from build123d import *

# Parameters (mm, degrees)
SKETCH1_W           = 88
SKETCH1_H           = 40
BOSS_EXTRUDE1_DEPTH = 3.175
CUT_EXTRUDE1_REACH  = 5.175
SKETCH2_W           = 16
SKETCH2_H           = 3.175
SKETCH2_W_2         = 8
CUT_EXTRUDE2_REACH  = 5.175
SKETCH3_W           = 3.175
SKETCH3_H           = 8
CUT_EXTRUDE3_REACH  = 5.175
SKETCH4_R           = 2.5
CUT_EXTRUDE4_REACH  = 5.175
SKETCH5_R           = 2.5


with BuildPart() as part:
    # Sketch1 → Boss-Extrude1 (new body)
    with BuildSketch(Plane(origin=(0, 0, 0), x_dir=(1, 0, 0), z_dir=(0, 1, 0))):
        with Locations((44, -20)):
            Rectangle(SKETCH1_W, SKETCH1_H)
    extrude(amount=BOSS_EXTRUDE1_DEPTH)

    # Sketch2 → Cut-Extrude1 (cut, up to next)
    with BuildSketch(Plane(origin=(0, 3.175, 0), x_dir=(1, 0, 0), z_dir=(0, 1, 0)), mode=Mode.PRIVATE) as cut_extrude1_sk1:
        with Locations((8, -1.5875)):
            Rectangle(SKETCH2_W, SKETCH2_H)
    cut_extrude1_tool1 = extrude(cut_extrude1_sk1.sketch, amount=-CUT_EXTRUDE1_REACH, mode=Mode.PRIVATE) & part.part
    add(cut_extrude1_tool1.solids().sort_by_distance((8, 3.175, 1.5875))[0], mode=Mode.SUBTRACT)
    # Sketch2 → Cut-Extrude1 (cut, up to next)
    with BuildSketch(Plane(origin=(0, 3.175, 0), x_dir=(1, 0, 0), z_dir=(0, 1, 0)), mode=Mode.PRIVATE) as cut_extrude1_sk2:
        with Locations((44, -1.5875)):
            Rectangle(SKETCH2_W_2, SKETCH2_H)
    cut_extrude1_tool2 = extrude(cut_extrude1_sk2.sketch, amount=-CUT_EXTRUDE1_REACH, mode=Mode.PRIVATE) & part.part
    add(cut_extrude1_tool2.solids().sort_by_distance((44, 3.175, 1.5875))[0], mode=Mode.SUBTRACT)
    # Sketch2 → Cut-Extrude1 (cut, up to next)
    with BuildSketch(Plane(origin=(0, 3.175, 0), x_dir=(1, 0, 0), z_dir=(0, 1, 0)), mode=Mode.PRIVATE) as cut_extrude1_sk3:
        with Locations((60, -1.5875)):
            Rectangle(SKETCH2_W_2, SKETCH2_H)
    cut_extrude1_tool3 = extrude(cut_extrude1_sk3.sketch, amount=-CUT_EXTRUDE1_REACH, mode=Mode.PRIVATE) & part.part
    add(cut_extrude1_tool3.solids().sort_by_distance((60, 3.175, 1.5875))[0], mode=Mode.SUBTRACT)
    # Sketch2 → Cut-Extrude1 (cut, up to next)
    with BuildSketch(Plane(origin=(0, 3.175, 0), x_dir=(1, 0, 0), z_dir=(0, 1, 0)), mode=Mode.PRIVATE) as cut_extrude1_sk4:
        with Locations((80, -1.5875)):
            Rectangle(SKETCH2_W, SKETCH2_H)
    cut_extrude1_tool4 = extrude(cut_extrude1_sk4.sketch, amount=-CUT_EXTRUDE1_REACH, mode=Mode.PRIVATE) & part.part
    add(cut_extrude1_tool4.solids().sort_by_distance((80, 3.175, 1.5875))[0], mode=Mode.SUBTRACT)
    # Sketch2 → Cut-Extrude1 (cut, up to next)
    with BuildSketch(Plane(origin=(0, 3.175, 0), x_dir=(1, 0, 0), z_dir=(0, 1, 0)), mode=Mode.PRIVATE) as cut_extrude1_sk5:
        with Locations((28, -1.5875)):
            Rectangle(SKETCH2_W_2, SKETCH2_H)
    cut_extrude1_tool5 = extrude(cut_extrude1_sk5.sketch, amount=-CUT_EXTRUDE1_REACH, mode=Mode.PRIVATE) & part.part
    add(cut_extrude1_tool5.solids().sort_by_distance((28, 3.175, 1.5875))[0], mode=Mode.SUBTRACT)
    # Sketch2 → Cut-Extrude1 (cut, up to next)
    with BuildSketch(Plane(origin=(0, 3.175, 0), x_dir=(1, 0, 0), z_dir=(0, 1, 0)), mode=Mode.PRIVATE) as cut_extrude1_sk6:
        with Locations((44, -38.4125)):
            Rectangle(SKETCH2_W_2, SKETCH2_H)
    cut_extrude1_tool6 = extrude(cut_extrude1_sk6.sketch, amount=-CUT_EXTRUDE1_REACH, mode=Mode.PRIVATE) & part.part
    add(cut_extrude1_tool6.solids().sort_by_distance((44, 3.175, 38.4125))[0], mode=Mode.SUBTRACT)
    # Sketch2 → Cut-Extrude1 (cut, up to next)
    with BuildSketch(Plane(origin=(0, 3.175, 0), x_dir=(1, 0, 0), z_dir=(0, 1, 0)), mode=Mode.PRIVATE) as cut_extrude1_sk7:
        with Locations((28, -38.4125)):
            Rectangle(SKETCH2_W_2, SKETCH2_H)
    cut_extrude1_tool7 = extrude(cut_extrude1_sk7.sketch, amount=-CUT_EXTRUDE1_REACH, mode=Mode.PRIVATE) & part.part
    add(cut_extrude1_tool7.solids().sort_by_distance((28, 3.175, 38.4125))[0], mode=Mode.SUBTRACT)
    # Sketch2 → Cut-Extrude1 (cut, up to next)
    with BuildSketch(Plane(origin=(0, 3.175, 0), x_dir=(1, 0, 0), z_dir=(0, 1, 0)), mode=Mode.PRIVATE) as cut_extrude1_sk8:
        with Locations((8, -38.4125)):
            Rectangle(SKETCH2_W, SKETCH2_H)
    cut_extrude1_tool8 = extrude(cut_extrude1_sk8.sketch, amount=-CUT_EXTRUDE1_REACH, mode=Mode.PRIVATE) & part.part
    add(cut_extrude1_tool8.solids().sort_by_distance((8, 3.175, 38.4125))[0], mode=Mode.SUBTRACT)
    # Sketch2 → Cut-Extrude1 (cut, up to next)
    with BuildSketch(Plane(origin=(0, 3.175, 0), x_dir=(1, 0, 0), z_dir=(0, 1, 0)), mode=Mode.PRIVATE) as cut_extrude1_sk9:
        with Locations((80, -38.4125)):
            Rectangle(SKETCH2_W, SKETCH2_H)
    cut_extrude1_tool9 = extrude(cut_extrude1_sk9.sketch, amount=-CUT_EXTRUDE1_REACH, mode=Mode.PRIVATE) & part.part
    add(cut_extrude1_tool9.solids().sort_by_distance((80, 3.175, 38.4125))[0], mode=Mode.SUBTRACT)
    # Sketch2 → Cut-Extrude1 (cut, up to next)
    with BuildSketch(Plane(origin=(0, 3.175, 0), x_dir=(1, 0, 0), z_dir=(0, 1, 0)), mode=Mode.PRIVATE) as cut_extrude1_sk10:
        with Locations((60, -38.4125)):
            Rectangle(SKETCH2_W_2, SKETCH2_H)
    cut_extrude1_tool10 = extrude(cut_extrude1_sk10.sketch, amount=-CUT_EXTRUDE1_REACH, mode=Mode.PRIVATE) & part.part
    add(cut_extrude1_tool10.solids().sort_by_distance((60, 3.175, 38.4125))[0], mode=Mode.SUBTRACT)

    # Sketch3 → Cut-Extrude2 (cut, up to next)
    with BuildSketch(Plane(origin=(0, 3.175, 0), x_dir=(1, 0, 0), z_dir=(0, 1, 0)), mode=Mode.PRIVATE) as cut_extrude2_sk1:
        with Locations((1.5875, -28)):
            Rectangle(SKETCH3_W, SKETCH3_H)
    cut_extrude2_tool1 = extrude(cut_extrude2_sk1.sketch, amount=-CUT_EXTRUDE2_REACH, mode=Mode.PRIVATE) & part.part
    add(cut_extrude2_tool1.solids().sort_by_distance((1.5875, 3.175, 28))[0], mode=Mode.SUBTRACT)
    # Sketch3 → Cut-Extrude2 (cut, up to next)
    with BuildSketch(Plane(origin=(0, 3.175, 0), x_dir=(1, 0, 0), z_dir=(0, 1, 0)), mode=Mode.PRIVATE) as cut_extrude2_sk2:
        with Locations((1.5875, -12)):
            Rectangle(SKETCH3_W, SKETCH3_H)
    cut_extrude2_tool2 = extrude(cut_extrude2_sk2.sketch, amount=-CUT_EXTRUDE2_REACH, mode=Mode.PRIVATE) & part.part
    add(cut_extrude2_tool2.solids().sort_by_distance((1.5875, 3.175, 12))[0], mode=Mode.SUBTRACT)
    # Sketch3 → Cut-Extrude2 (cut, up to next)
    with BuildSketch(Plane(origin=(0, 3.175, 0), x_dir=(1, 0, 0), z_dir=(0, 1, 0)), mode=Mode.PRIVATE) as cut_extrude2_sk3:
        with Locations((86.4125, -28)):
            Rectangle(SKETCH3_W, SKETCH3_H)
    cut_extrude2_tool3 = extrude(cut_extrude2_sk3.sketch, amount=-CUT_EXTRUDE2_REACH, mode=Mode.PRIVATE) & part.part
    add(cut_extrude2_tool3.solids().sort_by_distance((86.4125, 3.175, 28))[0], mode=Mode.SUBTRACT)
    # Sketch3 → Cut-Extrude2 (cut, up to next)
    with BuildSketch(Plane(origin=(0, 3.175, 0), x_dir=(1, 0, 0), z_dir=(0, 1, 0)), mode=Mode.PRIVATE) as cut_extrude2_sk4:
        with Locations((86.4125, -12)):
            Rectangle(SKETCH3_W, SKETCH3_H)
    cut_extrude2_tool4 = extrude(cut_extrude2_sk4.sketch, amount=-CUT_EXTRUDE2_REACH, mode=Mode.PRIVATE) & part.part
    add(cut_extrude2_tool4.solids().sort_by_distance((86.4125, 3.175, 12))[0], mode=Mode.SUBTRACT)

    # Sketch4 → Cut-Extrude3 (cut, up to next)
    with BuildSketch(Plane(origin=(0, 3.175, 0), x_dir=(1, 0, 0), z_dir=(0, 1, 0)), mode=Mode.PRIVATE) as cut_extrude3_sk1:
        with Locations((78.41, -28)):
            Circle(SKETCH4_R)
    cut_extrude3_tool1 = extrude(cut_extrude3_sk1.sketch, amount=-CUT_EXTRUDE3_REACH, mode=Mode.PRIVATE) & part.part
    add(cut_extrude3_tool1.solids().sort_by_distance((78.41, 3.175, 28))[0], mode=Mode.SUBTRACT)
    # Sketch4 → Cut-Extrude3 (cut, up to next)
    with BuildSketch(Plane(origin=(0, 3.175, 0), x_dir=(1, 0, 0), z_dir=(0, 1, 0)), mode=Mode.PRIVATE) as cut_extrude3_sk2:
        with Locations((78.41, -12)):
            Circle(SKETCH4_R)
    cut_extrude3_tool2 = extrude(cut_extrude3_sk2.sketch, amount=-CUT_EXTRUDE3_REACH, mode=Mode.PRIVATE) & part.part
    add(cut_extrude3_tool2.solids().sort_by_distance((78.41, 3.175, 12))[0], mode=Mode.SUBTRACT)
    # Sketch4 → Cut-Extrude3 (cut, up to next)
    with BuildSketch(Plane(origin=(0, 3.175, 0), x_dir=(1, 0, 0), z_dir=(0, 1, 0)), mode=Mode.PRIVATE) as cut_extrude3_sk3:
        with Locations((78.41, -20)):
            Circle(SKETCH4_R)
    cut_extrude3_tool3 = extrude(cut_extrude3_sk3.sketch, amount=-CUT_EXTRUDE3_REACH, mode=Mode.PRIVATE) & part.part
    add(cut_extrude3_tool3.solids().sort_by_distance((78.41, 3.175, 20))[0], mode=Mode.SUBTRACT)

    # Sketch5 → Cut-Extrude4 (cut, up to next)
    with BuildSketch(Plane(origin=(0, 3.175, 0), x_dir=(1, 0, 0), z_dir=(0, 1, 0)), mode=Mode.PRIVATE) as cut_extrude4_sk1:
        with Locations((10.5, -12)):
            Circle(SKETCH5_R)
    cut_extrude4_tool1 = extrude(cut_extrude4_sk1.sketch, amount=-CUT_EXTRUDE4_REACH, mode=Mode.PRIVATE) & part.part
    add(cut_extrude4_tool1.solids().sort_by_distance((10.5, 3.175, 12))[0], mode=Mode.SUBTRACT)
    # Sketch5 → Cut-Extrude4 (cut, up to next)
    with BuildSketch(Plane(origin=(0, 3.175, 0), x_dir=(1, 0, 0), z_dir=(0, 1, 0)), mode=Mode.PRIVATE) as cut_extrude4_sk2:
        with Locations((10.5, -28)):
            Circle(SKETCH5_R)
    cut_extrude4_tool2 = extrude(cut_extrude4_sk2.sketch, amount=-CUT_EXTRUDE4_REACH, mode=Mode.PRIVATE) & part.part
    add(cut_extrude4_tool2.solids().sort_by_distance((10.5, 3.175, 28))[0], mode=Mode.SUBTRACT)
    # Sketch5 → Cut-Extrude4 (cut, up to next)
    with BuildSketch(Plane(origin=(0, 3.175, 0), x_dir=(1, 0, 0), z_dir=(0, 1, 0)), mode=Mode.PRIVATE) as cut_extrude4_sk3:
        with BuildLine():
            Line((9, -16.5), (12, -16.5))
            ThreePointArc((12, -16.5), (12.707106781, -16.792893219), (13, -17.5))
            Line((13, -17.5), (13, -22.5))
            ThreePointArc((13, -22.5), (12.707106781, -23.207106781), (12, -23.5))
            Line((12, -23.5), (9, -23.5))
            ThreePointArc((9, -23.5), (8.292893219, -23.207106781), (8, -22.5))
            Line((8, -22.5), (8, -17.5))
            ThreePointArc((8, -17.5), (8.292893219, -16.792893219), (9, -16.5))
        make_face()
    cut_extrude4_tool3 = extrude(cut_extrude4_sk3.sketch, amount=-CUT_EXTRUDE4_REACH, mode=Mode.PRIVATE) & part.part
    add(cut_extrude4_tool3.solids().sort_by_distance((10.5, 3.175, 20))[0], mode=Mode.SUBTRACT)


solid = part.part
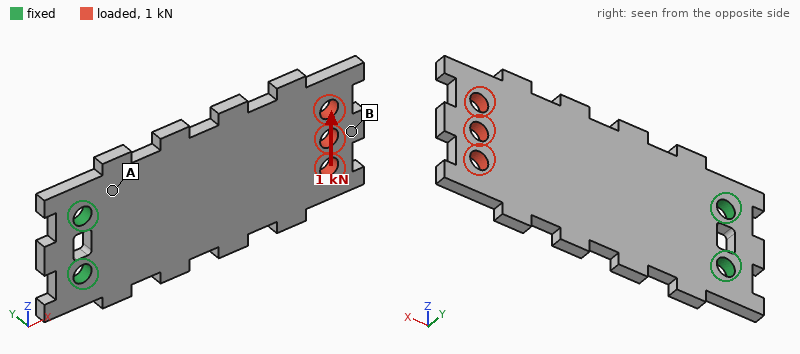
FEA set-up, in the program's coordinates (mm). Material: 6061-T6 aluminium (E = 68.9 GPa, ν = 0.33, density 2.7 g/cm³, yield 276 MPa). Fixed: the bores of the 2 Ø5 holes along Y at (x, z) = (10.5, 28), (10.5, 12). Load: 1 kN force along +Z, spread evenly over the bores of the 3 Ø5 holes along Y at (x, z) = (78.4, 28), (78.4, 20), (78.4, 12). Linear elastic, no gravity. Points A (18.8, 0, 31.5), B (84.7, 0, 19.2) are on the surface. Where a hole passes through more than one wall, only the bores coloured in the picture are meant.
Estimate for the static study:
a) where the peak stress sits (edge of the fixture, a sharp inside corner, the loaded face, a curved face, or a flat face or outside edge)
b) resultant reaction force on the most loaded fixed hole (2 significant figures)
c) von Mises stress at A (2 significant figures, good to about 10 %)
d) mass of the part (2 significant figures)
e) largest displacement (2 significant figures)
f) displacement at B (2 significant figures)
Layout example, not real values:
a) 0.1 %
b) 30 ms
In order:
a) edge of the fixture
b) 3.4 kN
c) 76 MPa
d) 25 g
e) 0.25 mm
f) 0.23 mm
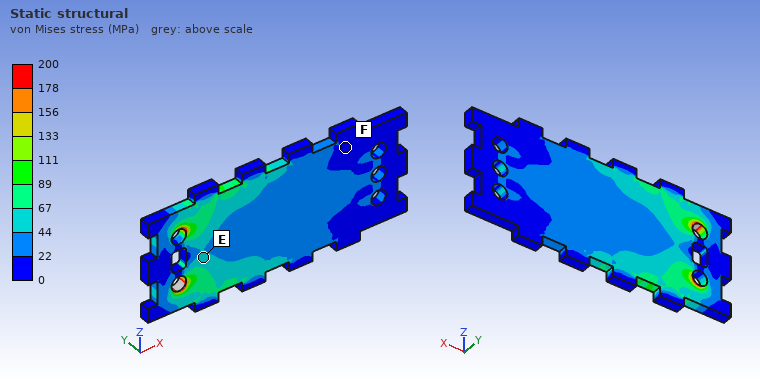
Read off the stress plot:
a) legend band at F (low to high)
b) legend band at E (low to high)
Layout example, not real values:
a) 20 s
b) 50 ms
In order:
a) 0 to 22 MPa
b) 44 to 67 MPa
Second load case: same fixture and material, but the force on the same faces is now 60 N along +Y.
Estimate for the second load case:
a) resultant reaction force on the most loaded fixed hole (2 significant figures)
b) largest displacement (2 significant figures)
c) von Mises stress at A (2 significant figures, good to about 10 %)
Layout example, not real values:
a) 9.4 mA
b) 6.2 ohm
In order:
a) 30 N
b) 1.1 mm
c) 58 MPa
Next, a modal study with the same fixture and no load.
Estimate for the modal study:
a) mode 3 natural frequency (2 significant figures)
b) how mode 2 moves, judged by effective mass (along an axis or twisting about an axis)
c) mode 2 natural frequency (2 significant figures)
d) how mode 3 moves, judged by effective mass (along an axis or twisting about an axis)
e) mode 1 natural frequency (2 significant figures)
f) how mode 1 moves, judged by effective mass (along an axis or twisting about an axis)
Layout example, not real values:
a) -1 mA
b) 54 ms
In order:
a) 2800 Hz
b) twisting about X
c) 1900 Hz
d) along Y
e) 470 Hz
f) along Y
